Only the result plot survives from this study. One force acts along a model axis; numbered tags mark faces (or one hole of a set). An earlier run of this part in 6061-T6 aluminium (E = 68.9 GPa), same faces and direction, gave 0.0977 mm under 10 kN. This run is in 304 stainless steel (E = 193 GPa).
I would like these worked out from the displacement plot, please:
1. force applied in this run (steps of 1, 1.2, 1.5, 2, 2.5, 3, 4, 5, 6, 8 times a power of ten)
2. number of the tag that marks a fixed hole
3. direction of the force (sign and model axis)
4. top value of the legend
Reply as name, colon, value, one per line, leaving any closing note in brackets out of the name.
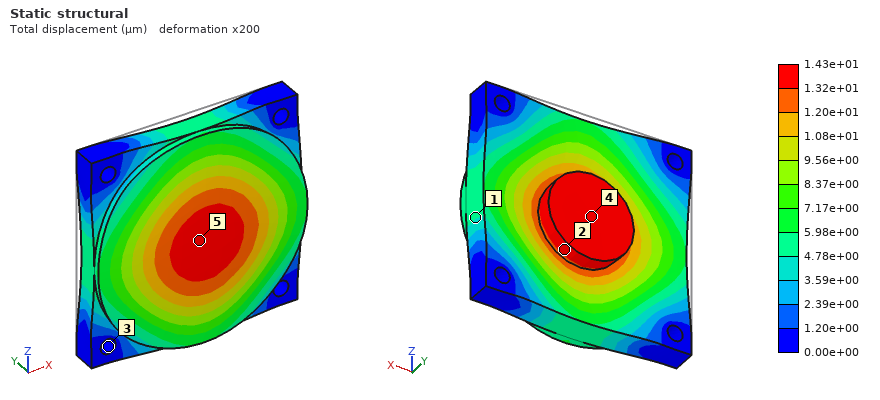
force applied in this run: 4 kN
number of the tag that marks a fixed hole: 3
direction of the force: -Y
top value of the legend: 1.43e+01 µm
